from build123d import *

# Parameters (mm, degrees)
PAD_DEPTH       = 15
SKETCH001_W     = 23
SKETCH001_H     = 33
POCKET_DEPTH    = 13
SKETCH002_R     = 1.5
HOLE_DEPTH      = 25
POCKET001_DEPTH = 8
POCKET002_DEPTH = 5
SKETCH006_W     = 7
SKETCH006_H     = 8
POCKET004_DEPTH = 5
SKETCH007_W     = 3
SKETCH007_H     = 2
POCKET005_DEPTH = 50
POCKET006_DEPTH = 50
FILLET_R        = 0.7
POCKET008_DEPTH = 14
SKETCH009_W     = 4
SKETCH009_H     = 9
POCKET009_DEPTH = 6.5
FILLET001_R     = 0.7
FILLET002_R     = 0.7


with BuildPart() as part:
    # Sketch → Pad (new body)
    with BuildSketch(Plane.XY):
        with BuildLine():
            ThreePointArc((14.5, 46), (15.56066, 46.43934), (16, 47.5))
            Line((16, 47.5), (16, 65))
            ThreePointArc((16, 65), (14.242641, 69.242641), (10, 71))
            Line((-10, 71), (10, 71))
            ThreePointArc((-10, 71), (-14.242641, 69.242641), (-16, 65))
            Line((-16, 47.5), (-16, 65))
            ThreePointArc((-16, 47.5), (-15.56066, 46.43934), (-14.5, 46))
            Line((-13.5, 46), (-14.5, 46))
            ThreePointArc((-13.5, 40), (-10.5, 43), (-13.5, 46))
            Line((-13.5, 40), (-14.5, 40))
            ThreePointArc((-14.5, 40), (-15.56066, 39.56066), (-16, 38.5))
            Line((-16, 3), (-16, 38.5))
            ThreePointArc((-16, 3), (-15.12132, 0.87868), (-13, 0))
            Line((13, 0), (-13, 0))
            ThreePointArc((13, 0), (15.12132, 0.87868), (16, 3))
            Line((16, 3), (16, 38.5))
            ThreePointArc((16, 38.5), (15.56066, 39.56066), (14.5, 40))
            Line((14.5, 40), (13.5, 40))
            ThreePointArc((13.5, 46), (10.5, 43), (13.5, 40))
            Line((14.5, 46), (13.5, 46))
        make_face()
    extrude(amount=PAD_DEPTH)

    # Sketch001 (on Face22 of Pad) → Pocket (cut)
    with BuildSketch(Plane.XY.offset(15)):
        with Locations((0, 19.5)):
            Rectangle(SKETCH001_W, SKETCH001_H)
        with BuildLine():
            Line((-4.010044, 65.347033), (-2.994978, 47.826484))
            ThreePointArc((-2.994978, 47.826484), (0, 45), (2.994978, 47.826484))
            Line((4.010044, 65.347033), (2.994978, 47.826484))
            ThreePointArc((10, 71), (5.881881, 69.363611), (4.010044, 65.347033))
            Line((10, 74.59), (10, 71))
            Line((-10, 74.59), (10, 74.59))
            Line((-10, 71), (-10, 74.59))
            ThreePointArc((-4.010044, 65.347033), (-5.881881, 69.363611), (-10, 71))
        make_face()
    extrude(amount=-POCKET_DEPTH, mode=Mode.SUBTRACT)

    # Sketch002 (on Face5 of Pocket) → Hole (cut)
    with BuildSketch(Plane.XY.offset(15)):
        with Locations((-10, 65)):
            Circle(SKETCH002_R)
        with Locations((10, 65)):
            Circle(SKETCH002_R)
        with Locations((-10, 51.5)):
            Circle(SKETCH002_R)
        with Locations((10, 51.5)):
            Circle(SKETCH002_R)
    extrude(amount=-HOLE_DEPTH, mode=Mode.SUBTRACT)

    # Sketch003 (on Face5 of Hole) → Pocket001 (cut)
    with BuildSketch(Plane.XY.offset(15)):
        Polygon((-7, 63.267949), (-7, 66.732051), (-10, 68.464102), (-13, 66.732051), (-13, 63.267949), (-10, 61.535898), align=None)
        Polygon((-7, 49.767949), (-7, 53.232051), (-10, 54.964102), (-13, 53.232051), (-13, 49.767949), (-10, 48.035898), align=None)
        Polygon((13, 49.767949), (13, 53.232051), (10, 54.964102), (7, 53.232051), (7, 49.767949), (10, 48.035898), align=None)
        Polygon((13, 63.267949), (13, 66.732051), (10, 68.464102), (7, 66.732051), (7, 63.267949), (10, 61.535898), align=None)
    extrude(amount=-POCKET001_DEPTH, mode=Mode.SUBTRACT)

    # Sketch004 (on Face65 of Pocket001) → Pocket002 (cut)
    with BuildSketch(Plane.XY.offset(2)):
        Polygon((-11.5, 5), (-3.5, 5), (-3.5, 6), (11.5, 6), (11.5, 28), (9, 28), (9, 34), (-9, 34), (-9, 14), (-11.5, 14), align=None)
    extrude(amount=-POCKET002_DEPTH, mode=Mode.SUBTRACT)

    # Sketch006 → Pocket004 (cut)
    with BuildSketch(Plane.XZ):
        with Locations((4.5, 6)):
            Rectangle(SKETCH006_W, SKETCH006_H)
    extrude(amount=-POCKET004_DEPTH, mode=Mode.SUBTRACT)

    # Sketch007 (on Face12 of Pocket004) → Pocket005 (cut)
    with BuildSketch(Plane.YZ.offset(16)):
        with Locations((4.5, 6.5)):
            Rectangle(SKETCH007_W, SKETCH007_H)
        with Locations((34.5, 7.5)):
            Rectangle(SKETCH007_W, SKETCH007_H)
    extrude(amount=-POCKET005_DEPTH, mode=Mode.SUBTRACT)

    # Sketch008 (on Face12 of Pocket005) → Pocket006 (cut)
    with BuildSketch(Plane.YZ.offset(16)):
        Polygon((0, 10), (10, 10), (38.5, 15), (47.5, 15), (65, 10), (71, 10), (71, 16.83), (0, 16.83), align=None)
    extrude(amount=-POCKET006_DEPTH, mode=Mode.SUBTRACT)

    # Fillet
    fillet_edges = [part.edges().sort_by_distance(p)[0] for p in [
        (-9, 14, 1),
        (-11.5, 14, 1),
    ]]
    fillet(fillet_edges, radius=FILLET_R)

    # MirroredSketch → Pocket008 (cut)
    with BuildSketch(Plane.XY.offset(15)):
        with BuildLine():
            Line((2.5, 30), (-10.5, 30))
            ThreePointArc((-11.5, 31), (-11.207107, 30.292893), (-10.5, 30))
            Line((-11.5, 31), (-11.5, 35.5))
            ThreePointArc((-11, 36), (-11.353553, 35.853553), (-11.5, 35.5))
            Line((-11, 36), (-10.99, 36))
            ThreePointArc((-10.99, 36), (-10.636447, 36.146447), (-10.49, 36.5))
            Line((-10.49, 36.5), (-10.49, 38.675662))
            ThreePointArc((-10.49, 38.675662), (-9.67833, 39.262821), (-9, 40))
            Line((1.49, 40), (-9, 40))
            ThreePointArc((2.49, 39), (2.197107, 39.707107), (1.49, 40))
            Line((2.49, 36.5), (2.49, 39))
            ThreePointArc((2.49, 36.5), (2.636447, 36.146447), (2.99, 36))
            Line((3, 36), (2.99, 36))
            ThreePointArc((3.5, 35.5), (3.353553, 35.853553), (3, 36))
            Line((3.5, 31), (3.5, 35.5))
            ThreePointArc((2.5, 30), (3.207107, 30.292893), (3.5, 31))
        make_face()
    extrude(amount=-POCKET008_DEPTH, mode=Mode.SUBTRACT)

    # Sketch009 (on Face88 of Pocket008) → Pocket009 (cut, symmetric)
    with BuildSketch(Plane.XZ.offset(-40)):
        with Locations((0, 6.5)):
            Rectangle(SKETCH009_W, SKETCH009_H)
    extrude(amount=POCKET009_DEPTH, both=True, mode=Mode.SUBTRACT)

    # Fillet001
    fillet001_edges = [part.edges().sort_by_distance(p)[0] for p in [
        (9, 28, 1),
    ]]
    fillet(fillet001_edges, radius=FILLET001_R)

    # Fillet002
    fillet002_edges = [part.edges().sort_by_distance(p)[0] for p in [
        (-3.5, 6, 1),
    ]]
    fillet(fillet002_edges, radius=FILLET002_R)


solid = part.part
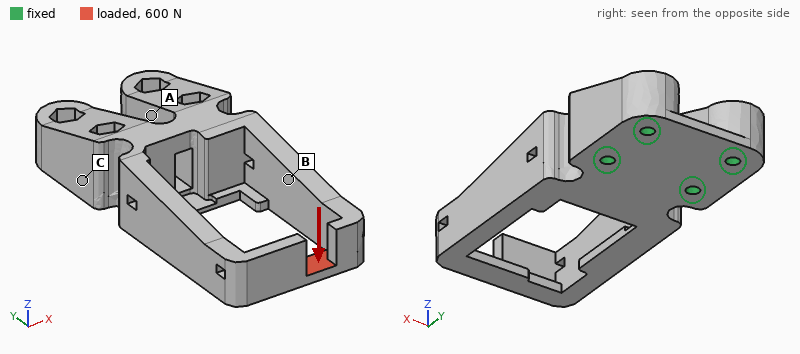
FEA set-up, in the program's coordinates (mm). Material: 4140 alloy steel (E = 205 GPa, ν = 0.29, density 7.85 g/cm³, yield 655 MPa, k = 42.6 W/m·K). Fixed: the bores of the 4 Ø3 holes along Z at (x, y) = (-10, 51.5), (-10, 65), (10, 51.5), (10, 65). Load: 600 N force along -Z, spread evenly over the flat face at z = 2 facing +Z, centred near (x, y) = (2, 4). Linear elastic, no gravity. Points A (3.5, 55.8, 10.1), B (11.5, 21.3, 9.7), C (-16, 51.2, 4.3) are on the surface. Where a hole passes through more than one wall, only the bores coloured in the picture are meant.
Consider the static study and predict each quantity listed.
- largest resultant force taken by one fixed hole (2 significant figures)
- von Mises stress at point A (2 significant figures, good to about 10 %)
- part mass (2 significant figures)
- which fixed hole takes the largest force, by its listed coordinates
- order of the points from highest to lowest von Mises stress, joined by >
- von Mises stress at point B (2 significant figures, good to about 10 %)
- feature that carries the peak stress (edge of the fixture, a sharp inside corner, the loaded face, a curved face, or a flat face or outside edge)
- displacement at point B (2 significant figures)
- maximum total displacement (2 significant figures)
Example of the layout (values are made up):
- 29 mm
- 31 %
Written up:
- 1.1 kN
- 37 MPa
- 110 g
- (10, 51.5)
- B > A > C
- 60 MPa
- a flat face or outside edge
- 0.042 mm
- 0.13 mm
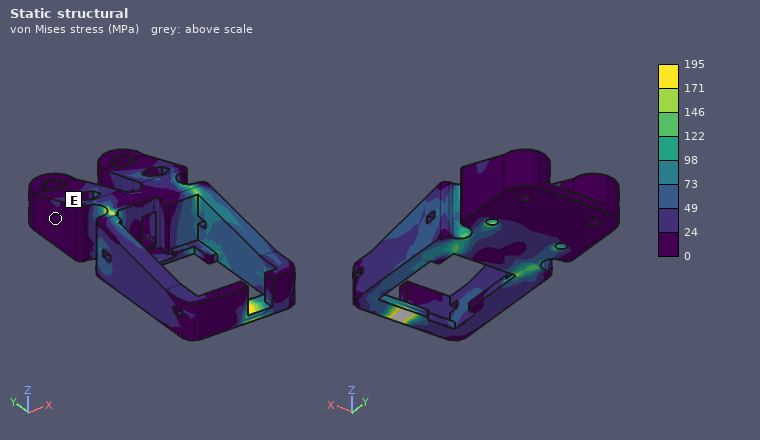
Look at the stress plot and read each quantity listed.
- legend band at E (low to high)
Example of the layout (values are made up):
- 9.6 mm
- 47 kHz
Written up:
- 0 to 24 MPa
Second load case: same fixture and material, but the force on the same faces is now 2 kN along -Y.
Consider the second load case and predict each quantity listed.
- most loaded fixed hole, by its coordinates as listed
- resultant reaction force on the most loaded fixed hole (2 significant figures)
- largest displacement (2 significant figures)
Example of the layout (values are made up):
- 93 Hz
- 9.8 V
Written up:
- (10, 51.5)
- 1.1 kN
- 70 µm
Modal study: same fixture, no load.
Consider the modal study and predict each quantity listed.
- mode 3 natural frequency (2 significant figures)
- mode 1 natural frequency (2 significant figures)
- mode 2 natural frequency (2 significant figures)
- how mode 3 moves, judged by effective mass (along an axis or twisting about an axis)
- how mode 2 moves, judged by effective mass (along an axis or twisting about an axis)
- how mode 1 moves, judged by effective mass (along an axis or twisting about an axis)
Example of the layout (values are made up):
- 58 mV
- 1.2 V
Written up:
- 5600 Hz
- 2500 Hz
- 3400 Hz
- twisting about Y
- along Z
- along X
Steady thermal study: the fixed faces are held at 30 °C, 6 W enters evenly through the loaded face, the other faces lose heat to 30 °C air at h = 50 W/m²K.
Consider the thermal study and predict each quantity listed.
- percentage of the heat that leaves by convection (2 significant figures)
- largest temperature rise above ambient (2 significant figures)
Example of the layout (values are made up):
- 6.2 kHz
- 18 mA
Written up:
- 62 %
- 58 K
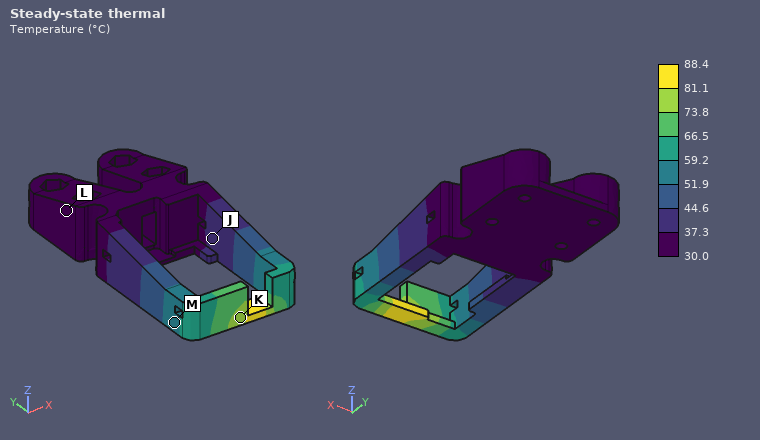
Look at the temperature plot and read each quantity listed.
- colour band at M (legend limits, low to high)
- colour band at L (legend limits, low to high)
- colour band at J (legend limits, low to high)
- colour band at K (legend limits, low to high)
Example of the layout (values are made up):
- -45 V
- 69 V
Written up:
- 51.9 to 59.2 °C
- 30.0 to 37.3 °C
- 37.3 to 44.6 °C
- 73.8 to 81.1 °C
